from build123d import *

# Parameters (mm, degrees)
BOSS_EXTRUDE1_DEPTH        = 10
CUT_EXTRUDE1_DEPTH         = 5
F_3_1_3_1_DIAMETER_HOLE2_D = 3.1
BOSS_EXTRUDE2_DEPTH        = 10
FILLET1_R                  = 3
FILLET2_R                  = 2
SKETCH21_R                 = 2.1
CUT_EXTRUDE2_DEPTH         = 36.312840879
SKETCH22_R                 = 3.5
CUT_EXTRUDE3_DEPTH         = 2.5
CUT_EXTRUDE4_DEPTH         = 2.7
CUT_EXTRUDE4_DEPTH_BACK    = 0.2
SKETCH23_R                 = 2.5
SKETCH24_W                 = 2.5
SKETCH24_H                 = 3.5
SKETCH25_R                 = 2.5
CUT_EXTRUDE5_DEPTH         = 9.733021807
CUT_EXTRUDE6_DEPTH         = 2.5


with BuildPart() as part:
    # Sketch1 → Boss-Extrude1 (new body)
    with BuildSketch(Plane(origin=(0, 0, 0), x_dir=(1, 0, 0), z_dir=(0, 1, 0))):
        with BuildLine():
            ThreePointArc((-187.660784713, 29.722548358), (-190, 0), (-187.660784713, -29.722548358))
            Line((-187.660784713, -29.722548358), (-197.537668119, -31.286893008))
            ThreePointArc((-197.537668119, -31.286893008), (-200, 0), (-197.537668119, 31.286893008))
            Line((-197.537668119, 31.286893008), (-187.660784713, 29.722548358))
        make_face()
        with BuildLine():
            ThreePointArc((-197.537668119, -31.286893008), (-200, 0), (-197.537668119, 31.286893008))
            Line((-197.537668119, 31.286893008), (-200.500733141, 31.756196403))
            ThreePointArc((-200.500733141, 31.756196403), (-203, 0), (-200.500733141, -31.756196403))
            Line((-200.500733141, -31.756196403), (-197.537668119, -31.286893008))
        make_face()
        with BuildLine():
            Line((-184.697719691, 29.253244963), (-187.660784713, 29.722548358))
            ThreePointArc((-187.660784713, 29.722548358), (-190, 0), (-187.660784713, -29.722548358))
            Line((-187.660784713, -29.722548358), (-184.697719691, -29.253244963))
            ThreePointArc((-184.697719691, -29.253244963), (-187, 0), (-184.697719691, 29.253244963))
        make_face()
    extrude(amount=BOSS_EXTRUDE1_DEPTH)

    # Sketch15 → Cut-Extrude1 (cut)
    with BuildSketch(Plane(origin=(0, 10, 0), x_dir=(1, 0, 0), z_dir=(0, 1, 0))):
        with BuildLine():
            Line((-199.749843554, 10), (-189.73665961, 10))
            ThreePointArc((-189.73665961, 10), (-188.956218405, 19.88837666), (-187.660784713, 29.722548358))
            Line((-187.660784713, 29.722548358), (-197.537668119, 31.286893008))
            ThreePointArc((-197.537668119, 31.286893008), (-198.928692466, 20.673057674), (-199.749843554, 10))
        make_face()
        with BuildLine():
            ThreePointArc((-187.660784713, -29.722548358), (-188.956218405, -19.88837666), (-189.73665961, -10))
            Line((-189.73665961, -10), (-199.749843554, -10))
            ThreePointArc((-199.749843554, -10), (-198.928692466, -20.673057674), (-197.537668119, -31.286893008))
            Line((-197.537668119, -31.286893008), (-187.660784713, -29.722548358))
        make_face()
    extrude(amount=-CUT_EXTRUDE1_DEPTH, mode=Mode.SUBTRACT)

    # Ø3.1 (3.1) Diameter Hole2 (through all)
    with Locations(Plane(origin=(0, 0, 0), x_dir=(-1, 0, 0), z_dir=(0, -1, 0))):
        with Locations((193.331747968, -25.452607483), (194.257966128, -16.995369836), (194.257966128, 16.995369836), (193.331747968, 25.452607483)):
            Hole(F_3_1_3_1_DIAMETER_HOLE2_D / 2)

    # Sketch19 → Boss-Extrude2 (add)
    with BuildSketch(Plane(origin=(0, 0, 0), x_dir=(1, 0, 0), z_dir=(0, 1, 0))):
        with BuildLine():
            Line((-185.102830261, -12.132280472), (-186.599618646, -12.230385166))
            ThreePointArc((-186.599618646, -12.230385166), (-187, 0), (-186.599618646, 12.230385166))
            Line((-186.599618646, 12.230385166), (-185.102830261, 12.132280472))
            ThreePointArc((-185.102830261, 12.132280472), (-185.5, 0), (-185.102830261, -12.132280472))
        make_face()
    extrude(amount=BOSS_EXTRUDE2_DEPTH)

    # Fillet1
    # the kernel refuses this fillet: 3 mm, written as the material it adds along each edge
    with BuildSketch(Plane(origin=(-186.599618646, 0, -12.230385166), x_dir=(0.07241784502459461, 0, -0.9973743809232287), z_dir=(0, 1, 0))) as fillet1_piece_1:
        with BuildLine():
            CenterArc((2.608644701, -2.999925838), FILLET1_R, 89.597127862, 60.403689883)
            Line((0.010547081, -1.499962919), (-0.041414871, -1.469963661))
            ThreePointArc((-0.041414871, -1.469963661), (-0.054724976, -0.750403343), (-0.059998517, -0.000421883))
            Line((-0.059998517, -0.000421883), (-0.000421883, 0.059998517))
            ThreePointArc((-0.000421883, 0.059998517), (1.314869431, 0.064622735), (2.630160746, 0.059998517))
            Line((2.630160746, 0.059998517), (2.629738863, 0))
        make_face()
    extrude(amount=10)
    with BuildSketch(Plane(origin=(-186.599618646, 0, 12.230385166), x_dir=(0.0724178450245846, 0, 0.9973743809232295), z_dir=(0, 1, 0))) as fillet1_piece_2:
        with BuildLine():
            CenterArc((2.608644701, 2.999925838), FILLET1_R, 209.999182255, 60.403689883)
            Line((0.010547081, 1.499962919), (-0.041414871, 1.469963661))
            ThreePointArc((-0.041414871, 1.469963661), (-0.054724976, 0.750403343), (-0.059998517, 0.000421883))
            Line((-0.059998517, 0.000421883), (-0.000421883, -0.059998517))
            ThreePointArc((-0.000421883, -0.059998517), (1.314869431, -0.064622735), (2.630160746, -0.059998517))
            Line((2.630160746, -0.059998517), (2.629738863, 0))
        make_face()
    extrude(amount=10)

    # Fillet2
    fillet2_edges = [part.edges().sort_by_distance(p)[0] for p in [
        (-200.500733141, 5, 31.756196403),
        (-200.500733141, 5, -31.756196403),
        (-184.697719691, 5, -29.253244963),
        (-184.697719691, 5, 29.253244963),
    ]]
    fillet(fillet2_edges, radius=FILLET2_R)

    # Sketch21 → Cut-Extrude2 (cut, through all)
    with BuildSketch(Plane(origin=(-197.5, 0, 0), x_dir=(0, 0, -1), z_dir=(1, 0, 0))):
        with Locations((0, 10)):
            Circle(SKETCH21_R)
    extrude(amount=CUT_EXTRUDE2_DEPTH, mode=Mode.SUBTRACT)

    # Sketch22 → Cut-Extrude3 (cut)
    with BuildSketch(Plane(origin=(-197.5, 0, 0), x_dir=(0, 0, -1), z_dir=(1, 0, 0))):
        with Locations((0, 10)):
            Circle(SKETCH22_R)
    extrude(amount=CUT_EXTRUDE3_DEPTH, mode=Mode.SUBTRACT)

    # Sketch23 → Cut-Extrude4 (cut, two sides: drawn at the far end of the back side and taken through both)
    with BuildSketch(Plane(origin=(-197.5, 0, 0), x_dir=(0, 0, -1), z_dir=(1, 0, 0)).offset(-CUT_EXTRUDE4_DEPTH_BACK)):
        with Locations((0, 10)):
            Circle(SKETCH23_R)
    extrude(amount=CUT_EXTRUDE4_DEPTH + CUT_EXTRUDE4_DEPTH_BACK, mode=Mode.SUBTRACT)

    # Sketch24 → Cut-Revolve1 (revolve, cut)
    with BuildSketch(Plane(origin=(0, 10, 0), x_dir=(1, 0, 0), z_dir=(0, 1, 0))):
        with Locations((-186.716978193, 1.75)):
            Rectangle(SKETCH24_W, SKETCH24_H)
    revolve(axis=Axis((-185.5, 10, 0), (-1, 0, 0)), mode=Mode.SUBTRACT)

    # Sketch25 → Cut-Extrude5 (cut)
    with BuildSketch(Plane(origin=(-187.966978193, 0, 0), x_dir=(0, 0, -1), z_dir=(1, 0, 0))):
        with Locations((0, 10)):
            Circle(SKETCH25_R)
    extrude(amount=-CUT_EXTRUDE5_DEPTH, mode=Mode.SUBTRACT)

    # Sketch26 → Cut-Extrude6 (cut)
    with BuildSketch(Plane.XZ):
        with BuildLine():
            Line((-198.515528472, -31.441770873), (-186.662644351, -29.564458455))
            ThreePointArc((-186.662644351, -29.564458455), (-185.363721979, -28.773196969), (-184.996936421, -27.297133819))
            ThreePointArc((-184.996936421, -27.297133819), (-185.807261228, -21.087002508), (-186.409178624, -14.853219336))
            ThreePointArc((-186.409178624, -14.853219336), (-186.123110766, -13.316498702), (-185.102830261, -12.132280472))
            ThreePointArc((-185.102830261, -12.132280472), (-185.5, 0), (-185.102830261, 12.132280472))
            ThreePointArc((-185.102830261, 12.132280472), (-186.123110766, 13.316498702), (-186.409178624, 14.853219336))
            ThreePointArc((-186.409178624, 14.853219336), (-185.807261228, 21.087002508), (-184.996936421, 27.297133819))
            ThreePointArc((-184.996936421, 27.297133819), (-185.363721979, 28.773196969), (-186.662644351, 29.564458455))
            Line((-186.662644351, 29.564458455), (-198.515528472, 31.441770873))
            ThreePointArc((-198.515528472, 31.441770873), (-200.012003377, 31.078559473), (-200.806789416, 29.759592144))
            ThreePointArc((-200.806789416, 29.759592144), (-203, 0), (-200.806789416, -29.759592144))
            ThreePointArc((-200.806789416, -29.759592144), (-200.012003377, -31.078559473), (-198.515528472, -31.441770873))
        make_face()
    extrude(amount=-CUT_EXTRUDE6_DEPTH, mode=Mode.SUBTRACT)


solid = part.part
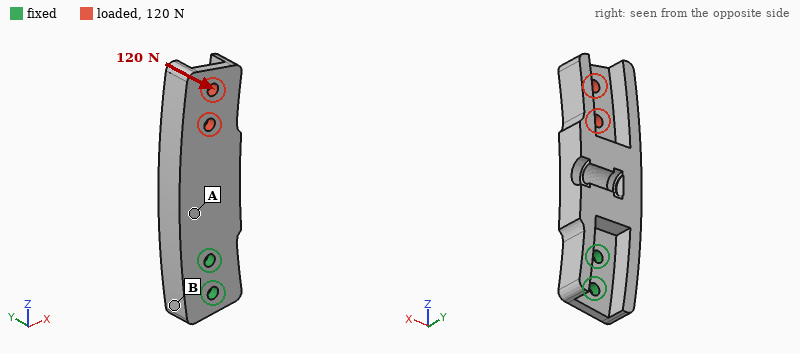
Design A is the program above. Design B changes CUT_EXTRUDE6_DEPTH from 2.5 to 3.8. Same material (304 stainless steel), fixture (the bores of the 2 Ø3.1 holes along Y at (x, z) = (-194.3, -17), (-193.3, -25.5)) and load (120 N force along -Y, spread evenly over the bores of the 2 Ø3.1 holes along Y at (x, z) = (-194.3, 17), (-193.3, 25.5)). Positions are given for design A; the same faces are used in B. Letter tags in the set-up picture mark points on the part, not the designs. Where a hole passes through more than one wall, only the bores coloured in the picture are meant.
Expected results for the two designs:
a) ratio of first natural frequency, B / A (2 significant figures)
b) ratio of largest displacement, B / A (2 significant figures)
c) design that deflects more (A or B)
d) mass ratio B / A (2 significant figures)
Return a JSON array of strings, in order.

["0.68", "2.7", "B", "0.76"]
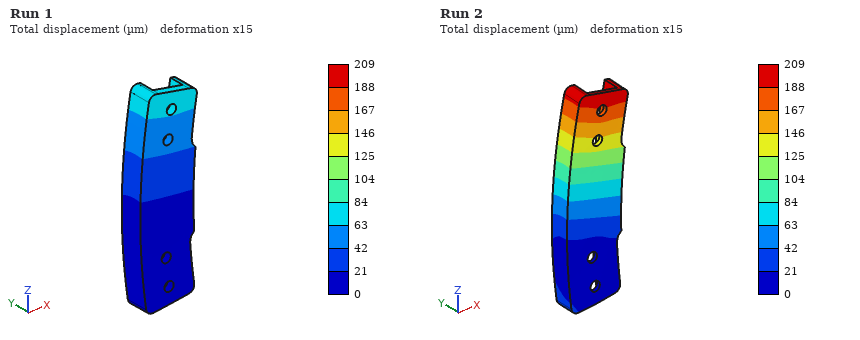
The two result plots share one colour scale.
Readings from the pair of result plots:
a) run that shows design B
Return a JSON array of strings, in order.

["Run 2"]
